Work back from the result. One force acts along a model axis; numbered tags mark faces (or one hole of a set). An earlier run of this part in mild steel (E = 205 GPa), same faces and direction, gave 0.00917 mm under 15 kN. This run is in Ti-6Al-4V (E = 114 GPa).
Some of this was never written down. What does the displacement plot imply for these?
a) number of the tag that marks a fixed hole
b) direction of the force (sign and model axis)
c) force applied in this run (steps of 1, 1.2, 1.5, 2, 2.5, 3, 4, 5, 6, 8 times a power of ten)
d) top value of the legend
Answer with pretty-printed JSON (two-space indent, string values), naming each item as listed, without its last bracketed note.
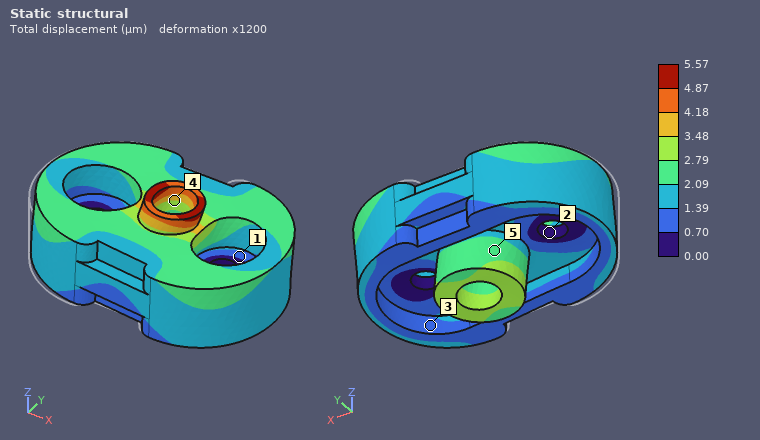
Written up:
{
  "number of the tag that marks a fixed hole": "2",
  "direction of the force": "+X",
  "force applied in this run": "5 kN",
  "top value of the legend": "5.57 µm"
}
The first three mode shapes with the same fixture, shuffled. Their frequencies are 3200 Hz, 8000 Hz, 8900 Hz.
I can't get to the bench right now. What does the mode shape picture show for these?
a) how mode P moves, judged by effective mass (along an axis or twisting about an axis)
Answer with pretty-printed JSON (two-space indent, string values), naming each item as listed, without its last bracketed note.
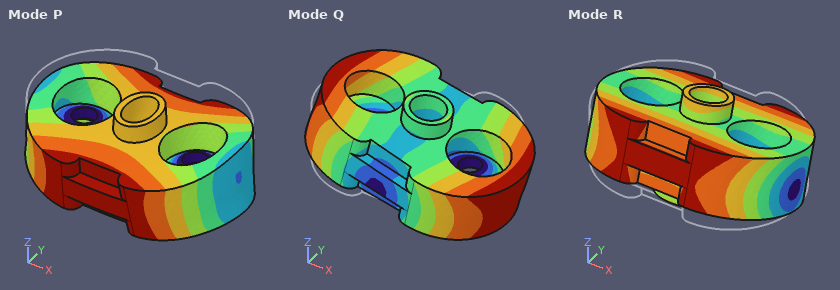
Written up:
{
  "how mode P moves, judged by effective mass": "along Z"
}
